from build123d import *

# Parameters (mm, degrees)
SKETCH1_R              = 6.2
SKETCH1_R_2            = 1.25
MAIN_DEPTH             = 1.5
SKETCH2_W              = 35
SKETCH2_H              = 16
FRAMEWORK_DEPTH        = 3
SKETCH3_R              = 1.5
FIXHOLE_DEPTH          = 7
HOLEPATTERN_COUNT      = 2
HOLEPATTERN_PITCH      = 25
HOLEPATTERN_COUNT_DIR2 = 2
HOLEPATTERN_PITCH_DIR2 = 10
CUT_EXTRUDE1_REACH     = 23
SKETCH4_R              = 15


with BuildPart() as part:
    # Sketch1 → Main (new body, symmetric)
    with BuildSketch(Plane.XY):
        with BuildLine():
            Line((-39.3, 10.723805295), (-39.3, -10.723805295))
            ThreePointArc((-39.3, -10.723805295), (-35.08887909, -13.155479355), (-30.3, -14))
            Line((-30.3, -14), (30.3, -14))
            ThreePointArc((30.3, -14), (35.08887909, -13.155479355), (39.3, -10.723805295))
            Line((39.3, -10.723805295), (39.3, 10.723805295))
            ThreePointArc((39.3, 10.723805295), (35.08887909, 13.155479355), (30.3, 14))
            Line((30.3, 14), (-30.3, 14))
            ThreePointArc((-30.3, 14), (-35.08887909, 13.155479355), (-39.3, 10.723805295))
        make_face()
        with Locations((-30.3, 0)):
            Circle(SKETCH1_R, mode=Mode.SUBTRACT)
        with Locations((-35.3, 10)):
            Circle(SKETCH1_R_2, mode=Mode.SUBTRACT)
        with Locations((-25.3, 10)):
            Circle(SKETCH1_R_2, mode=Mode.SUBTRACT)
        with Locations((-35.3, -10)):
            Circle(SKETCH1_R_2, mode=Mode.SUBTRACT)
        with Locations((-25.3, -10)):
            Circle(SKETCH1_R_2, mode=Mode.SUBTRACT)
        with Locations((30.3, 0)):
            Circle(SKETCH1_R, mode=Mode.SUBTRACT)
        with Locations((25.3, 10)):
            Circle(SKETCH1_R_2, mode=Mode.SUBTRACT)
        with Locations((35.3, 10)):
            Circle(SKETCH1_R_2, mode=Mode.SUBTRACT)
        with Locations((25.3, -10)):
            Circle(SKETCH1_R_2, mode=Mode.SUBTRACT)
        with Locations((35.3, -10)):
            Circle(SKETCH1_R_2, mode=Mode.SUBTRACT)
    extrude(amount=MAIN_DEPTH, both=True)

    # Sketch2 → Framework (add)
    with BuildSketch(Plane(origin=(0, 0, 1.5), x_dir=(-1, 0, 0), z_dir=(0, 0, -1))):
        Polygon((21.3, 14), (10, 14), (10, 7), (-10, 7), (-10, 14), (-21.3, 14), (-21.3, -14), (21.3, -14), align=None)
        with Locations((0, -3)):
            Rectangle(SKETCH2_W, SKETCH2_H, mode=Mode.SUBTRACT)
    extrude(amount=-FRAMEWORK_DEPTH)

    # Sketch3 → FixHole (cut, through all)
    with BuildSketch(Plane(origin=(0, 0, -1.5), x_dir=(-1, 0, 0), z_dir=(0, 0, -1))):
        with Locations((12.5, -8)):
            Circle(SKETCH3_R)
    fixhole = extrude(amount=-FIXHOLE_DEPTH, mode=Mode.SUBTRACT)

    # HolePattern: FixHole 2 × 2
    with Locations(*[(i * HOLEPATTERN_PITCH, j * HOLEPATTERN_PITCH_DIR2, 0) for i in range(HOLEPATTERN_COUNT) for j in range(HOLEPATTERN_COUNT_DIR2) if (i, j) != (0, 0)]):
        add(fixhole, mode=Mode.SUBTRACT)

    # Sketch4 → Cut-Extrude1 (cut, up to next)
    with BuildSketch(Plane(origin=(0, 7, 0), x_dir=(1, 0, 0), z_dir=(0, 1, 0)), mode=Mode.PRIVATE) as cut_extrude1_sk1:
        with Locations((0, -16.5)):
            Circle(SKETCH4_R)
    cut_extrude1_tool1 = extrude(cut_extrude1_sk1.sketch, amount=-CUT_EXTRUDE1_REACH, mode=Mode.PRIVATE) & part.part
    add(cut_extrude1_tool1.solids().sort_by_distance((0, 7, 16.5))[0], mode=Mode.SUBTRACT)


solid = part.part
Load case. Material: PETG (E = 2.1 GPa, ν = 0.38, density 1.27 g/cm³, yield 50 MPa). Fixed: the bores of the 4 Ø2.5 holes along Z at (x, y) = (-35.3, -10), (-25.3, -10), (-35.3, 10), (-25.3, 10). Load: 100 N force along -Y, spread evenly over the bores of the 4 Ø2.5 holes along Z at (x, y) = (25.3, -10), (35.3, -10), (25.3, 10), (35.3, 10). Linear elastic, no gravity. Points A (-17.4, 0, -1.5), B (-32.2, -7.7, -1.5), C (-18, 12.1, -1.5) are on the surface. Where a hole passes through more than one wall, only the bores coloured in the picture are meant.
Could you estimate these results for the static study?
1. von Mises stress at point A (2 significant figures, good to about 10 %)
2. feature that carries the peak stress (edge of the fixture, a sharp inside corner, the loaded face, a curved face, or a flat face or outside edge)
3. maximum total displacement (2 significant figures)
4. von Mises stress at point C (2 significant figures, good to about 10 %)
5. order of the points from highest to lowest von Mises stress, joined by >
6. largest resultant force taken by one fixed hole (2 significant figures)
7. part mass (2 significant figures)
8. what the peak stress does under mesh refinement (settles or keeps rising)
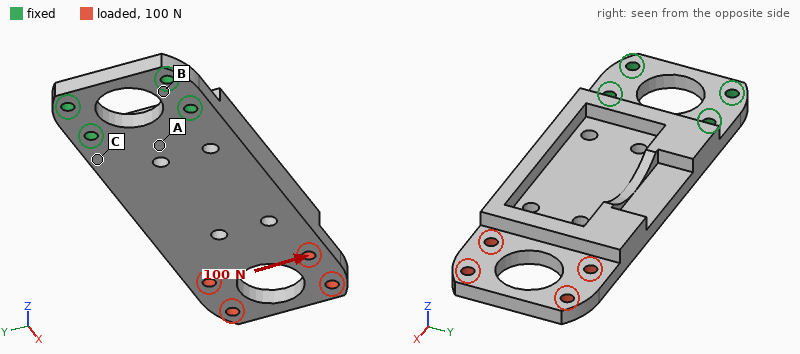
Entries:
4.1 MPa
edge of the fixture
0.84 mm
11 MPa
C > A > B
240 N
8.8 g
keeps rising
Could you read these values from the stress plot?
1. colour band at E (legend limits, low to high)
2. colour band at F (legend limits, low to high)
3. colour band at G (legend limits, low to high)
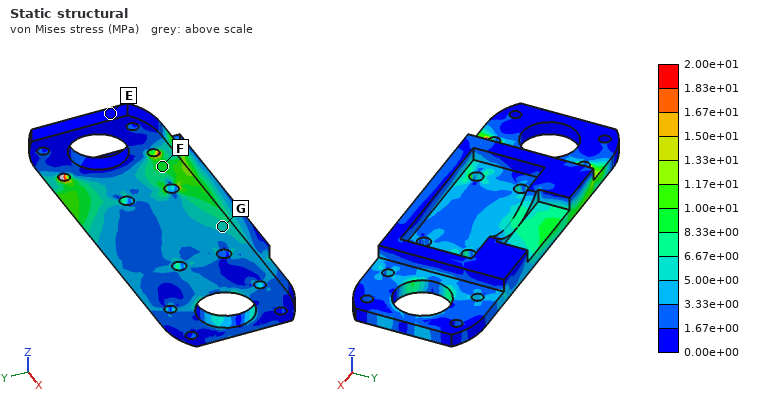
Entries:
0.00e+00 to 1.67e+00 MPa
8.33e+00 to 1.00e+01 MPa
5.00e+00 to 6.67e+00 MPa
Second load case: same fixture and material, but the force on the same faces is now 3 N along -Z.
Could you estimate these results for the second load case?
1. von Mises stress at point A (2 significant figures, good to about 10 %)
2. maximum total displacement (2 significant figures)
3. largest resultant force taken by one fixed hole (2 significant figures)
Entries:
1.1 MPa
0.97 mm
4.6 N
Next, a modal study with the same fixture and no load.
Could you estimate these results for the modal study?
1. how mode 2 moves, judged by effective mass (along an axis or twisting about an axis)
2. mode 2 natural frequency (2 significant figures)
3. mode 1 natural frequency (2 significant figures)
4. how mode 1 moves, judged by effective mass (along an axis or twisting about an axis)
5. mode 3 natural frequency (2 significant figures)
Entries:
twisting about X
800 Hz
200 Hz
along Z
1100 Hz
